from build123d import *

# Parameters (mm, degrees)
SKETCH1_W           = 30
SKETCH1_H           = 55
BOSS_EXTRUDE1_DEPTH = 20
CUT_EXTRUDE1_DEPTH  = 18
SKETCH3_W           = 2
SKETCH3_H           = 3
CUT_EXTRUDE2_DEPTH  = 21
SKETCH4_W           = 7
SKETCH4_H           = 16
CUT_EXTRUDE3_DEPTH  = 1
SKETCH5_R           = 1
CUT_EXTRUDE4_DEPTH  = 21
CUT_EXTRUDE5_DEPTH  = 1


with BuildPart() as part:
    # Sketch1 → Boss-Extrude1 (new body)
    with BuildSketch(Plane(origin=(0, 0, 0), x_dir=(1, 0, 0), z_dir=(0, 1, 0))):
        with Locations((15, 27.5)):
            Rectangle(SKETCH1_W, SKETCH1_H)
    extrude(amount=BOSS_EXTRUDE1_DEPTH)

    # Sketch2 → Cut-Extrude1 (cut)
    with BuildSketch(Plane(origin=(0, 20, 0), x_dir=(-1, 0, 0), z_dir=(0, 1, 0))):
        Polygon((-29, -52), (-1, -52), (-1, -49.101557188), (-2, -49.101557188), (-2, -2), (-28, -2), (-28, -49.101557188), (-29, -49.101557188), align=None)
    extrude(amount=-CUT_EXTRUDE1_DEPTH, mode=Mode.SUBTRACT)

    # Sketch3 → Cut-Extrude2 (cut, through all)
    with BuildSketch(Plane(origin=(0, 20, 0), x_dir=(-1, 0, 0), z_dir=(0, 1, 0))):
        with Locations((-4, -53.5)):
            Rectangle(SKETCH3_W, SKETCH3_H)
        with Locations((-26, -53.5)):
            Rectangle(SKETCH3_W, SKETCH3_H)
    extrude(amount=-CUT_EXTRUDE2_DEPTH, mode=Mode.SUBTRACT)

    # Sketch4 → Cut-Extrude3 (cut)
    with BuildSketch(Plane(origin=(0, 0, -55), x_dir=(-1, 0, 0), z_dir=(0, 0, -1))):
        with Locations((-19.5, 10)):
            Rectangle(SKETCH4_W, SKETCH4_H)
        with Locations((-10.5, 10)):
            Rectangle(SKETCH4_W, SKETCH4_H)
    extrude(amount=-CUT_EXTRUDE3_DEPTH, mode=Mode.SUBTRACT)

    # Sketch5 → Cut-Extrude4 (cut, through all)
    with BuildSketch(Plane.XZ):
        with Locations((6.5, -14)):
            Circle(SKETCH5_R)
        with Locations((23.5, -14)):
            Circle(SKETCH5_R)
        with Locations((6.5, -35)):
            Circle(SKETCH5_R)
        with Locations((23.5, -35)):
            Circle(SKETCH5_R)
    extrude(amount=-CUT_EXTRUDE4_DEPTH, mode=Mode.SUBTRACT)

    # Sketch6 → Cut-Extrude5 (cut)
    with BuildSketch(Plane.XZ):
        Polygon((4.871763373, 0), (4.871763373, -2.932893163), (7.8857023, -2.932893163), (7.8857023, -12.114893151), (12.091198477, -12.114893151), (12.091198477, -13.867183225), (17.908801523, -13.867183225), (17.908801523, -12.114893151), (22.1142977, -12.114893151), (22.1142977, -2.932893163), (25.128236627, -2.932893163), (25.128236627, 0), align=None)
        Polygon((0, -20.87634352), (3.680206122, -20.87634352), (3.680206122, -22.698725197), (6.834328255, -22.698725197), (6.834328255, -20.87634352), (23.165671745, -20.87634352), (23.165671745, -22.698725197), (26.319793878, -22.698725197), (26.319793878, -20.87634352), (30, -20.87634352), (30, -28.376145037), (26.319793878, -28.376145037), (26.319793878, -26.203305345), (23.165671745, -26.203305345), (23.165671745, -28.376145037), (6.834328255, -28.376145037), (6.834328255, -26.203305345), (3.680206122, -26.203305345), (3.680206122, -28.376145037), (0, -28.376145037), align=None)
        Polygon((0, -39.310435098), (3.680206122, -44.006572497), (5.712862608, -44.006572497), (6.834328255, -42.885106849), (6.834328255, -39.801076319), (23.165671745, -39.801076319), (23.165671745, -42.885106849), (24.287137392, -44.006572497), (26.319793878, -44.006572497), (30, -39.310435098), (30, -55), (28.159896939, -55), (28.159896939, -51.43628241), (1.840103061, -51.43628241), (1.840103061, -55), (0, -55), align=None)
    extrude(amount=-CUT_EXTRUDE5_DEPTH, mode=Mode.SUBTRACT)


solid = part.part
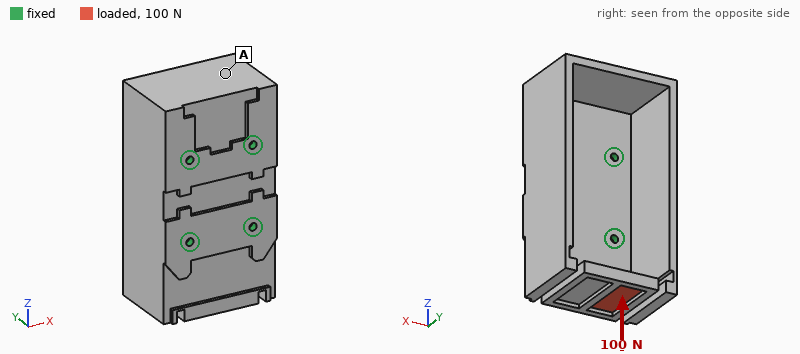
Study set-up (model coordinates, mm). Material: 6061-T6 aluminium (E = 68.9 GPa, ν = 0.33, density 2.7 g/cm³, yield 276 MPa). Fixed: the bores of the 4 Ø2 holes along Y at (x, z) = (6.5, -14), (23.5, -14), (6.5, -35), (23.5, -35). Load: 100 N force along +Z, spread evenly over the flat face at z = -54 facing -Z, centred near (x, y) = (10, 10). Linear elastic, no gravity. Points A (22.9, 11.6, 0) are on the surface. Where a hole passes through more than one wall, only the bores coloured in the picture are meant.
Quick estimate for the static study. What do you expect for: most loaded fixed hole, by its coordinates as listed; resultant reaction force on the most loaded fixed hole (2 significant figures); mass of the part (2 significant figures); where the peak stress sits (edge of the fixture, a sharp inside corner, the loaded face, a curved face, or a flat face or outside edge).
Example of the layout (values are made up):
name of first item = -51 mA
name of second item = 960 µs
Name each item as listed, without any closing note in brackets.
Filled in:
most loaded fixed hole, by its coordinates as listed = (6.5, -35)
resultant reaction force on the most loaded fixed hole = 62 N
mass of the part = 22 g
where the peak stress sits = a flat face or outside edge
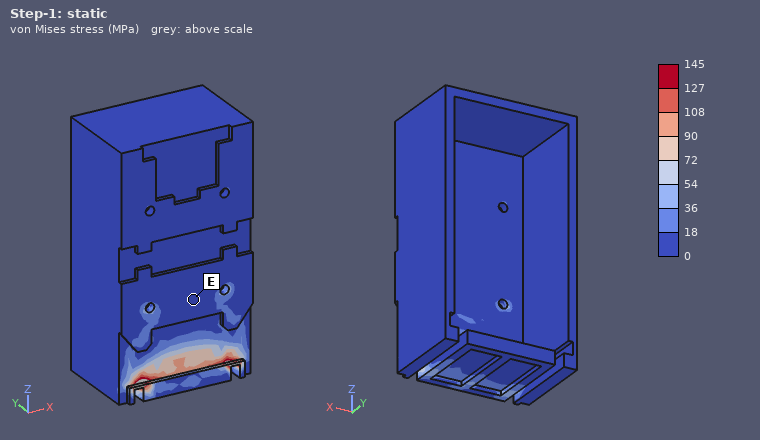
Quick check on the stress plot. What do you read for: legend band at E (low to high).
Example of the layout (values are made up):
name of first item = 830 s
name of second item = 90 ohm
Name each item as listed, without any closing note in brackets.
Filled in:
legend band at E = 0 to 18 MPa
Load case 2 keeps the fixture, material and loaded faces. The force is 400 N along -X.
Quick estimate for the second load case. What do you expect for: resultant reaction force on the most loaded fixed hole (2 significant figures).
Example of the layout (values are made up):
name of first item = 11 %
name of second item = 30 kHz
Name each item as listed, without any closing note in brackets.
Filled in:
resultant reaction force on the most loaded fixed hole = 480 N
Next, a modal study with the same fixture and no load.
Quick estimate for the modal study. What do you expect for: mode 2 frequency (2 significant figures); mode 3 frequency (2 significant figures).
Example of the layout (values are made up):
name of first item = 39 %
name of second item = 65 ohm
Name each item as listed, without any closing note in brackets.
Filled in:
mode 2 frequency = 2900 Hz
mode 3 frequency = 3000 Hz
